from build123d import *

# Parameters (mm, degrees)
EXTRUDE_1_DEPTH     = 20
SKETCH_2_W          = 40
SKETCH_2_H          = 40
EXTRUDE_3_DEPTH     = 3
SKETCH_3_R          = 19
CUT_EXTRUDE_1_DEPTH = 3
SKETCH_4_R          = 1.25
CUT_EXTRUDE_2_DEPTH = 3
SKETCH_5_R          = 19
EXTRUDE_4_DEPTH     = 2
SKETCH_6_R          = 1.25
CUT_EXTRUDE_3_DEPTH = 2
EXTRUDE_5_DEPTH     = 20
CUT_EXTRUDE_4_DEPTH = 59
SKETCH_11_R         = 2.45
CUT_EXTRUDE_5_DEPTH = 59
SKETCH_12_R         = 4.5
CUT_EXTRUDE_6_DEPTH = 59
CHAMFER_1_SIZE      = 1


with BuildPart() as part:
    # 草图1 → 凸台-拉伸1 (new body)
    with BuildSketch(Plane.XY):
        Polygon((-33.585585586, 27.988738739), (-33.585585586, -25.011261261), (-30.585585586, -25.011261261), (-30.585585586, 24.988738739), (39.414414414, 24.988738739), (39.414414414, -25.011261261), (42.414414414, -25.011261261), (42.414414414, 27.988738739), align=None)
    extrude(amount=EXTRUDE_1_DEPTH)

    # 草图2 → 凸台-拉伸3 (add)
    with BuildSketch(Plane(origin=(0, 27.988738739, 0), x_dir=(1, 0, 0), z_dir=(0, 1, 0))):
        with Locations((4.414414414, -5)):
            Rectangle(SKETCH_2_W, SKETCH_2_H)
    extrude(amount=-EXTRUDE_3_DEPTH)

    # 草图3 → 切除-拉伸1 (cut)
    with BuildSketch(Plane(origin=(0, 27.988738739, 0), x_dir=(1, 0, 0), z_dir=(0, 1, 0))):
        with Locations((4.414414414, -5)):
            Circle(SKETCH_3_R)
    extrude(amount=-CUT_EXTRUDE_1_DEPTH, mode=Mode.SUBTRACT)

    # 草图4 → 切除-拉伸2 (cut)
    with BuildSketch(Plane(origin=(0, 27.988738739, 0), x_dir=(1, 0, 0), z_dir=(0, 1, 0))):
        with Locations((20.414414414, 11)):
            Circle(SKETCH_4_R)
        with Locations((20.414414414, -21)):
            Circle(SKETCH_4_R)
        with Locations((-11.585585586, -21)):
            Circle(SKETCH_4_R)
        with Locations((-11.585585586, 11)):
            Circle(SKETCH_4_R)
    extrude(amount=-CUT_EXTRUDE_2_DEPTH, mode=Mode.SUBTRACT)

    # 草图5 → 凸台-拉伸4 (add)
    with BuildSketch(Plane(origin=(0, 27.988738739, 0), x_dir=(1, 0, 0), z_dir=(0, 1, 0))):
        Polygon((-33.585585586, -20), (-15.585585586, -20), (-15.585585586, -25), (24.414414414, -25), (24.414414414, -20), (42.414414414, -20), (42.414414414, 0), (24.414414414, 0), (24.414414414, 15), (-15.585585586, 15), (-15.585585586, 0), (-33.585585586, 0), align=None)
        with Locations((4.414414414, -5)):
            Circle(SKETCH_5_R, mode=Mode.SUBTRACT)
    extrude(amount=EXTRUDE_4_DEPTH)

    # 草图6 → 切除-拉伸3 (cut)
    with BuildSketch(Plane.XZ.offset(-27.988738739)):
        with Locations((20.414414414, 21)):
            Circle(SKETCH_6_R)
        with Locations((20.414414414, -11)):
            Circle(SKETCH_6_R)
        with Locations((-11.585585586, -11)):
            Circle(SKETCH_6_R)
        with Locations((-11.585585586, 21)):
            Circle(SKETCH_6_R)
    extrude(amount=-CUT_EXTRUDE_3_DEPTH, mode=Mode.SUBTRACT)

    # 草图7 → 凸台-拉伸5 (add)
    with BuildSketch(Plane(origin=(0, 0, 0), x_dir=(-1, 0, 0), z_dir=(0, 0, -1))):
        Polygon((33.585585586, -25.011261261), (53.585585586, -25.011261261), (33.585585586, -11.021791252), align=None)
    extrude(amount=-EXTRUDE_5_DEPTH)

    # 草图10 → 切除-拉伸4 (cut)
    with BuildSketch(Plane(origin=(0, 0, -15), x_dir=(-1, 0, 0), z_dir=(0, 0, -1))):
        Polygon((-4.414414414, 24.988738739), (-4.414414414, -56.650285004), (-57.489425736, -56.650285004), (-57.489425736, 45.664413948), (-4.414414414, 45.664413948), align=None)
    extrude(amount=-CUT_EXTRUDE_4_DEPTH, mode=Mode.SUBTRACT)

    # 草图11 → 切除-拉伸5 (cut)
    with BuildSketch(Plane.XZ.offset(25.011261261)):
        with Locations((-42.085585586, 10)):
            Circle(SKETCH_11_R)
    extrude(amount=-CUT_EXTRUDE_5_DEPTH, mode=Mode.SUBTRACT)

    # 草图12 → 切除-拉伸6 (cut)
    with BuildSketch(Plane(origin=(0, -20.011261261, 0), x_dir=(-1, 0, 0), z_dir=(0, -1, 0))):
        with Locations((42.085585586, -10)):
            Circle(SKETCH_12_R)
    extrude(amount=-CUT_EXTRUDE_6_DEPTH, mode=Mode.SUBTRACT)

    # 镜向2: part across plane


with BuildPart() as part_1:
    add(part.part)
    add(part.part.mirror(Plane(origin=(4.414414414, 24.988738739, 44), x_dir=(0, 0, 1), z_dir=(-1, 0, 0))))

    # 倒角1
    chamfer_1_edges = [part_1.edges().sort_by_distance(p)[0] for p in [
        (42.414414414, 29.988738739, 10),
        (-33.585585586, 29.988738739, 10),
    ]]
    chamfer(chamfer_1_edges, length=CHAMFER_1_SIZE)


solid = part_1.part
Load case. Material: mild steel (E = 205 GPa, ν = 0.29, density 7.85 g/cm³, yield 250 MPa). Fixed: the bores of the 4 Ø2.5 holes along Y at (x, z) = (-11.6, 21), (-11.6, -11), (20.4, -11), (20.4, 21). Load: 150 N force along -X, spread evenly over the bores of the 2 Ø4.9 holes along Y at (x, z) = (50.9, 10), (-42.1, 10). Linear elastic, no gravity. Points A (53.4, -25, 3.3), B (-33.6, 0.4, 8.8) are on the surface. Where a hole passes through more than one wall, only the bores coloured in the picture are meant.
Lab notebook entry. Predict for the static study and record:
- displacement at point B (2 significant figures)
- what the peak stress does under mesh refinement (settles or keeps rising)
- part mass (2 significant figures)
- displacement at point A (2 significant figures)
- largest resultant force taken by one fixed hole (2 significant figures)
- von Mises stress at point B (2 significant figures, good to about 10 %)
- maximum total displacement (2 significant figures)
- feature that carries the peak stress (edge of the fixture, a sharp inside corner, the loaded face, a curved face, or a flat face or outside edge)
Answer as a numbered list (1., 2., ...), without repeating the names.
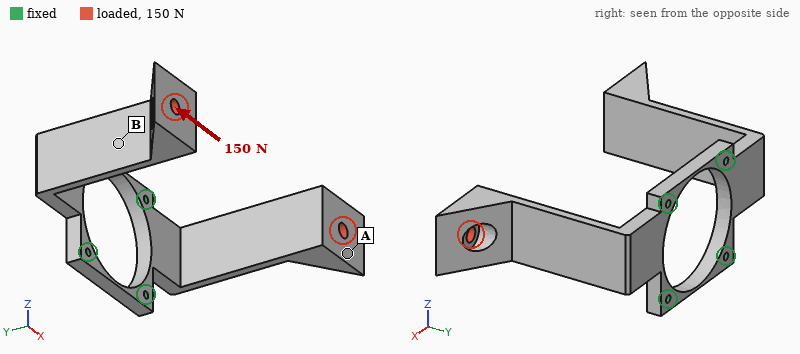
1. 0.20 mm
2. keeps rising
3. 130 g
4. 0.53 mm
5. 64 N
6. 55 MPa
7. 0.58 mm
8. edge of the fixture
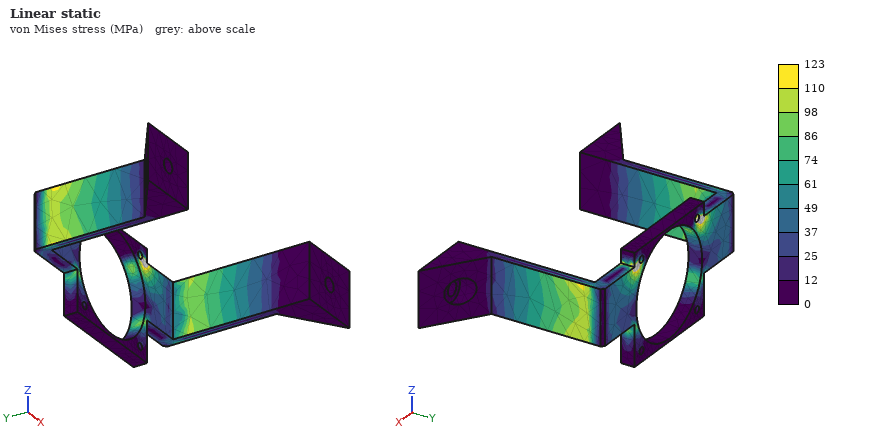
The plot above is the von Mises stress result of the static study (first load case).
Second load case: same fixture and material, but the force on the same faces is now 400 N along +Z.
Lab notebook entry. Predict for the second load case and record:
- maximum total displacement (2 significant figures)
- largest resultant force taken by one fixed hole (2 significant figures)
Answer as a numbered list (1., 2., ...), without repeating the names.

1. 0.31 mm
2. 520 N
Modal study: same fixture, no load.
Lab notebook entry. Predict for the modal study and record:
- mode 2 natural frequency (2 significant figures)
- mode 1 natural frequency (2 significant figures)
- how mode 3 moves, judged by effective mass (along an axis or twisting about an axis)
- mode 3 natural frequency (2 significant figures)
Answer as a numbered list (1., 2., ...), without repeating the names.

1. 380 Hz
2. 380 Hz
3. along Z
4. 920 Hz
